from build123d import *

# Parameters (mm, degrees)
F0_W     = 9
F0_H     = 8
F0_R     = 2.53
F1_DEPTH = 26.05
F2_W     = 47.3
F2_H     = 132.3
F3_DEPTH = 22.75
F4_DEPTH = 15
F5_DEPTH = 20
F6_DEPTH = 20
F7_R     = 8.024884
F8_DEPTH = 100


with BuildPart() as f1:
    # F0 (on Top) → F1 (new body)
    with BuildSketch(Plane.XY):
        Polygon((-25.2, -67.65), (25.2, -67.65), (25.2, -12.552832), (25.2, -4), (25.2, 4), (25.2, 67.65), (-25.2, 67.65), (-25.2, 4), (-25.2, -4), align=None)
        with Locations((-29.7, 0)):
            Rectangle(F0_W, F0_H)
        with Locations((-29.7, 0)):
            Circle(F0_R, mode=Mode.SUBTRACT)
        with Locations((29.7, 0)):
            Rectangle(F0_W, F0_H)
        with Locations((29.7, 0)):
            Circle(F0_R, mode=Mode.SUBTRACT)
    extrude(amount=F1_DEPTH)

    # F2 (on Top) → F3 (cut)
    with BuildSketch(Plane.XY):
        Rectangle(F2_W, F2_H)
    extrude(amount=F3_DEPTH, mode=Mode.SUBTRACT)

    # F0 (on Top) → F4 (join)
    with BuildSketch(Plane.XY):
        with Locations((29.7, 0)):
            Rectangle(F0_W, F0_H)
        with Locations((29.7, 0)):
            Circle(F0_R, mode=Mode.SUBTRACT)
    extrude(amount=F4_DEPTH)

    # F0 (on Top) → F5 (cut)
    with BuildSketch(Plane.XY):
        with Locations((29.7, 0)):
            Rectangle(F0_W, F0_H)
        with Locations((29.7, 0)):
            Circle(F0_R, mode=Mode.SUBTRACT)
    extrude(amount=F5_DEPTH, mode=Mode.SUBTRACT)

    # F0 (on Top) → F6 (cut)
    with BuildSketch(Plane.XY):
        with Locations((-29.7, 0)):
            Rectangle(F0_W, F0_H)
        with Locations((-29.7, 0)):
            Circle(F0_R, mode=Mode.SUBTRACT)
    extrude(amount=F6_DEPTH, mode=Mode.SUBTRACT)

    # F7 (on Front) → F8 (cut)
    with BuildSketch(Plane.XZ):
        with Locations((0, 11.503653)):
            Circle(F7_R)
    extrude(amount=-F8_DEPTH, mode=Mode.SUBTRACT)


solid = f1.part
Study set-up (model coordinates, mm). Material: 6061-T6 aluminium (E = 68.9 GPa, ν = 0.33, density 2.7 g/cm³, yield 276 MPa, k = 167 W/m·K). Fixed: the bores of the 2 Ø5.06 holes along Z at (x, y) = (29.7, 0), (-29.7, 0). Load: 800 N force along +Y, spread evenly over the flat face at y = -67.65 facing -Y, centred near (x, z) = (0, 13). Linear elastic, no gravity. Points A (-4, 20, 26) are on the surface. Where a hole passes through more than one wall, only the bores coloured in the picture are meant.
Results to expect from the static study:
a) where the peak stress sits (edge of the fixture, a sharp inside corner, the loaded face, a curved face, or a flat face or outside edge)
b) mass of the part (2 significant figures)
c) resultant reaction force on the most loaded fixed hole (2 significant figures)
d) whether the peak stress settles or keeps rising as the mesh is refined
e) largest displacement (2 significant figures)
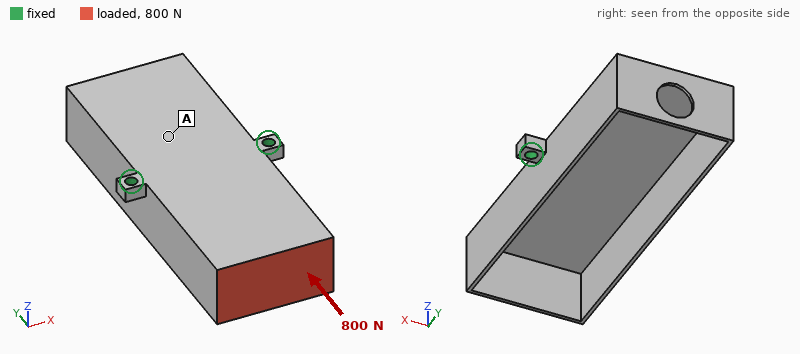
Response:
edge of the fixture
96 g
400 N
keeps rising
0.50 mm
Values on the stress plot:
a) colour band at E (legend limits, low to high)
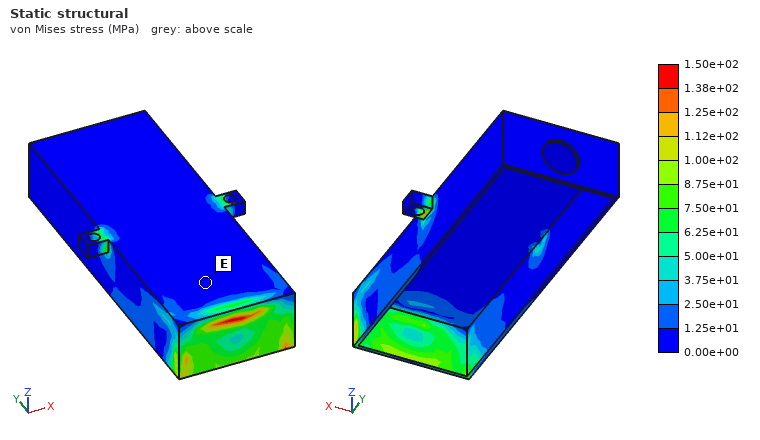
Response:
0.00e+00 to 1.25e+01 MPa
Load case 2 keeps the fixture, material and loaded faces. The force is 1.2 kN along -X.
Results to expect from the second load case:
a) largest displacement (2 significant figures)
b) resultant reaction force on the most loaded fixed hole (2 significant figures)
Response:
0.75 mm
1.7 kN
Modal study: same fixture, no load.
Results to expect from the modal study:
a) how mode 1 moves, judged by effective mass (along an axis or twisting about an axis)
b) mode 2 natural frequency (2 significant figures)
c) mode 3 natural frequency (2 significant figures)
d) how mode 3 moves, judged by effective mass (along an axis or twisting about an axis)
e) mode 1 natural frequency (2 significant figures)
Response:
twisting about X
1200 Hz
2500 Hz
along Z
720 Hz
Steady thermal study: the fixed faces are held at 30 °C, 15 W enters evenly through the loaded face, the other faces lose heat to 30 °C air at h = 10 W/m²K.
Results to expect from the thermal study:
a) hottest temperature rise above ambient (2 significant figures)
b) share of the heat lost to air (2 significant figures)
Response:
35 K
21 %
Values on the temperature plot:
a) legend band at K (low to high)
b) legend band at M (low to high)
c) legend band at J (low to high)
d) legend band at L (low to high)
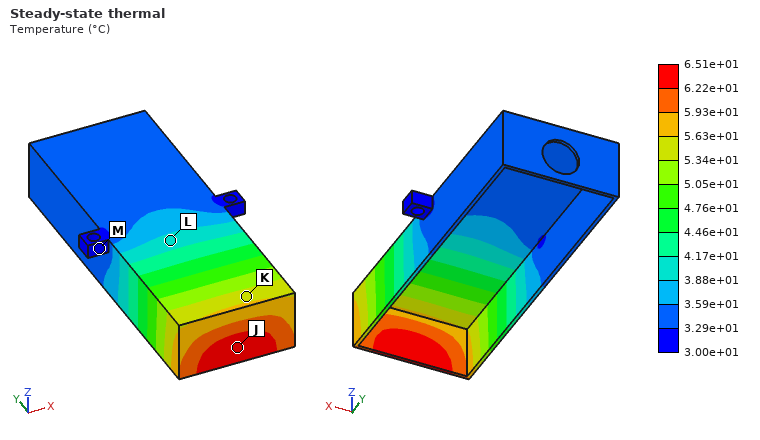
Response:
5.34e+01 to 5.63e+01 °C
3.00e+01 to 3.29e+01 °C
6.22e+01 to 6.51e+01 °C
3.88e+01 to 4.17e+01 °C
